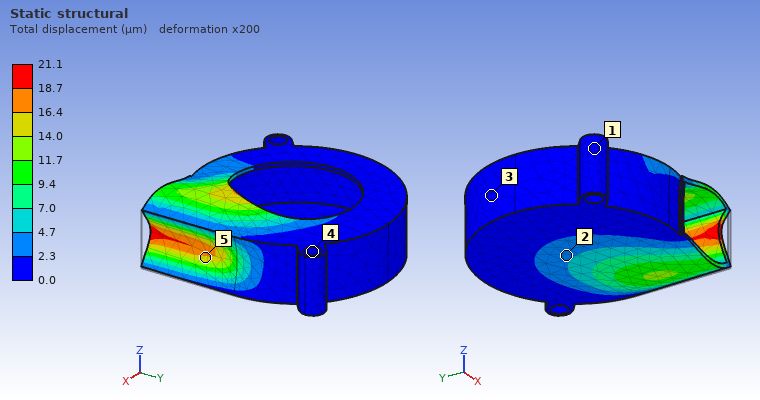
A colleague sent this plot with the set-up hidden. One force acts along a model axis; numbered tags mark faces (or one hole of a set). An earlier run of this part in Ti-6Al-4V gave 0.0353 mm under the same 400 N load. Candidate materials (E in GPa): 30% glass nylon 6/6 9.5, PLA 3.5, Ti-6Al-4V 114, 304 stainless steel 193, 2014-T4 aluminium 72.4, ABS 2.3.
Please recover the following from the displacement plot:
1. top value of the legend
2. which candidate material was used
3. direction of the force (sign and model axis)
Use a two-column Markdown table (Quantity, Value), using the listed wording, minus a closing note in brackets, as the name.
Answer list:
| Quantity | Value |
|---|---|
| top value of the legend | 21.1 µm |
| which candidate material was used | 304 stainless steel |
| direction of the force | -X |
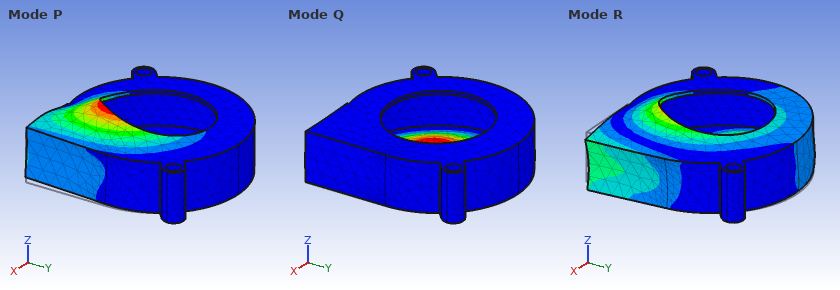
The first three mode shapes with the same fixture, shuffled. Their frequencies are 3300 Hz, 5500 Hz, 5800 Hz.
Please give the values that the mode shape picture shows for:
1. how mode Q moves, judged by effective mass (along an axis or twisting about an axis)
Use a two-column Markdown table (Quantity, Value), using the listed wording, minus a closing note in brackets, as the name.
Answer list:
| Quantity | Value |
|---|---|
| how mode Q moves, judged by effective mass | along Z |
